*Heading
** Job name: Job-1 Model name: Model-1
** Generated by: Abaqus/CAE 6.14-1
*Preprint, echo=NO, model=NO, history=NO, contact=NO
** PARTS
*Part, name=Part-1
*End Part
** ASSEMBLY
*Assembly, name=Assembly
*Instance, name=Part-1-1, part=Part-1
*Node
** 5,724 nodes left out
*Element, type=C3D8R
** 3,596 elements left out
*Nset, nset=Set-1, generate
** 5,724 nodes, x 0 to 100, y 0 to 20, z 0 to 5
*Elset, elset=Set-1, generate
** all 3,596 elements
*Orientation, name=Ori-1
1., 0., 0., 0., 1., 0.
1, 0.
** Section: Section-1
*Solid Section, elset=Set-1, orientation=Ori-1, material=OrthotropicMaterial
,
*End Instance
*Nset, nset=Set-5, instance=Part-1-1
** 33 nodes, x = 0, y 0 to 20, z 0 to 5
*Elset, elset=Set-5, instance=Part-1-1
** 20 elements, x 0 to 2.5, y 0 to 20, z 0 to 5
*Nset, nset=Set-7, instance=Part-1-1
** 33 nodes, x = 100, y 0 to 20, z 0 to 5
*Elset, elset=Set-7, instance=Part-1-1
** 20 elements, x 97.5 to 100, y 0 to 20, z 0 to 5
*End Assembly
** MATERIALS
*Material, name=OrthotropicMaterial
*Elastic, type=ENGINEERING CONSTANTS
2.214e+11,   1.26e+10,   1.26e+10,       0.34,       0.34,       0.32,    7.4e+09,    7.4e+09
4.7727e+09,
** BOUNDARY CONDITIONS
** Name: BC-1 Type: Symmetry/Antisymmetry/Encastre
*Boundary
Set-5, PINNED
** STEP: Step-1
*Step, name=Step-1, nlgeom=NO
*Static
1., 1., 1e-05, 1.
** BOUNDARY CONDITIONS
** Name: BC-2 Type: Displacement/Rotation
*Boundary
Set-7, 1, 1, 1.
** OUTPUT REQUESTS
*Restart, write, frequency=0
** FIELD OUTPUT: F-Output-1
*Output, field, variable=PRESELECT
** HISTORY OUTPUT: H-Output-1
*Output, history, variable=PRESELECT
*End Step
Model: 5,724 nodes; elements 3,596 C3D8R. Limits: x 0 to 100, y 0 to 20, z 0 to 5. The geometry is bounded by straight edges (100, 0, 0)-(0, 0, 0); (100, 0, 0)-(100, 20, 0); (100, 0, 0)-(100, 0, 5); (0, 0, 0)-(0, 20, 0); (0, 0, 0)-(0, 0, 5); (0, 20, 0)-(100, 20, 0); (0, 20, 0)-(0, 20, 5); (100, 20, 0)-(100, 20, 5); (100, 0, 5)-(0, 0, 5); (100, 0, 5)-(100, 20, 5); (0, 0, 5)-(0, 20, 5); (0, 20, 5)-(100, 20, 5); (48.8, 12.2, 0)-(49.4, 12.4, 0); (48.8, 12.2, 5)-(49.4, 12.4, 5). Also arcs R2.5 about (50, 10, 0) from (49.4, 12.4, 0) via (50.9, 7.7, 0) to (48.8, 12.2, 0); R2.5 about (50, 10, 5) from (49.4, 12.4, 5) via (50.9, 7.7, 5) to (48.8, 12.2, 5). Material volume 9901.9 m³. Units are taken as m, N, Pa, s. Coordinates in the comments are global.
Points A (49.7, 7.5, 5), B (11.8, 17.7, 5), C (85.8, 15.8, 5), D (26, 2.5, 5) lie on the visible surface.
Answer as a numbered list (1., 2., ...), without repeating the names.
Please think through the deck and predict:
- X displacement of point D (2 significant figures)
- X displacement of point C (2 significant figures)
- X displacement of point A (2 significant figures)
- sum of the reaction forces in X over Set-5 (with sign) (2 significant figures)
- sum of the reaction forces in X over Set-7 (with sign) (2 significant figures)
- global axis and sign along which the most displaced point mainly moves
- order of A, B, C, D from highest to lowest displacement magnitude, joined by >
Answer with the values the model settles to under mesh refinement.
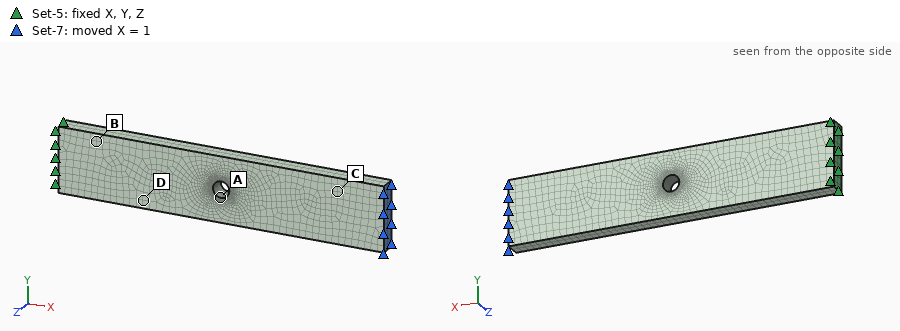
1. 0.25 m
2. 0.87 m
3. 0.48 m
4. -2.1e+11 N
5. 2.1e+11 N
6. +X
7. C > A > D > B
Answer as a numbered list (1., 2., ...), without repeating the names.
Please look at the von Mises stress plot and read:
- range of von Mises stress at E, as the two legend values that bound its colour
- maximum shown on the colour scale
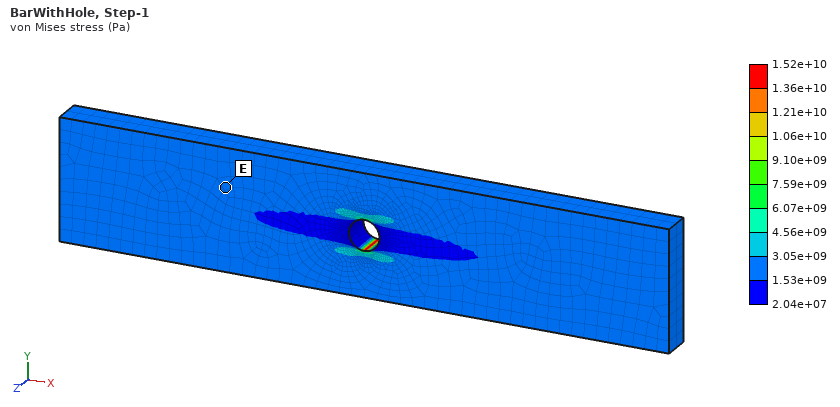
1. 1.53e+09 to 3.05e+09 Pa
2. 1.52e+10 Pa
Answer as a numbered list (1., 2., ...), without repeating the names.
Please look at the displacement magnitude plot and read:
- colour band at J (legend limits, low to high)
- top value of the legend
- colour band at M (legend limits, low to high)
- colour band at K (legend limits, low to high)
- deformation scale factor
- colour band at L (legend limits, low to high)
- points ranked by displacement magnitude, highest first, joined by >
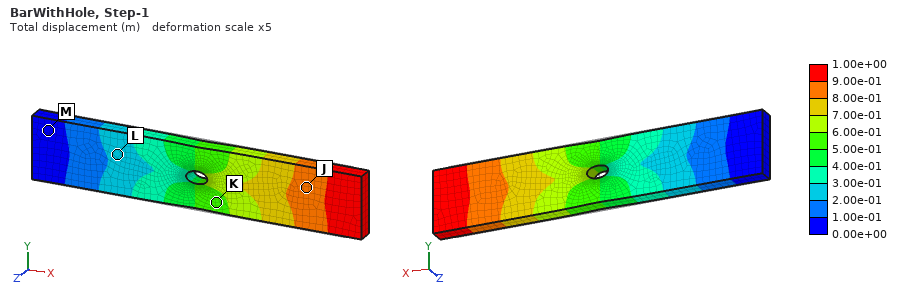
1. 8.00e-01 to 9.00e-01 m
2. 1.00e+00 m
3. 0.00e+00 to 1.00e-01 m
4. 5.00e-01 to 6.00e-01 m
5. 5
6. 2.00e-01 to 3.00e-01 m
7. J > K > L > M
